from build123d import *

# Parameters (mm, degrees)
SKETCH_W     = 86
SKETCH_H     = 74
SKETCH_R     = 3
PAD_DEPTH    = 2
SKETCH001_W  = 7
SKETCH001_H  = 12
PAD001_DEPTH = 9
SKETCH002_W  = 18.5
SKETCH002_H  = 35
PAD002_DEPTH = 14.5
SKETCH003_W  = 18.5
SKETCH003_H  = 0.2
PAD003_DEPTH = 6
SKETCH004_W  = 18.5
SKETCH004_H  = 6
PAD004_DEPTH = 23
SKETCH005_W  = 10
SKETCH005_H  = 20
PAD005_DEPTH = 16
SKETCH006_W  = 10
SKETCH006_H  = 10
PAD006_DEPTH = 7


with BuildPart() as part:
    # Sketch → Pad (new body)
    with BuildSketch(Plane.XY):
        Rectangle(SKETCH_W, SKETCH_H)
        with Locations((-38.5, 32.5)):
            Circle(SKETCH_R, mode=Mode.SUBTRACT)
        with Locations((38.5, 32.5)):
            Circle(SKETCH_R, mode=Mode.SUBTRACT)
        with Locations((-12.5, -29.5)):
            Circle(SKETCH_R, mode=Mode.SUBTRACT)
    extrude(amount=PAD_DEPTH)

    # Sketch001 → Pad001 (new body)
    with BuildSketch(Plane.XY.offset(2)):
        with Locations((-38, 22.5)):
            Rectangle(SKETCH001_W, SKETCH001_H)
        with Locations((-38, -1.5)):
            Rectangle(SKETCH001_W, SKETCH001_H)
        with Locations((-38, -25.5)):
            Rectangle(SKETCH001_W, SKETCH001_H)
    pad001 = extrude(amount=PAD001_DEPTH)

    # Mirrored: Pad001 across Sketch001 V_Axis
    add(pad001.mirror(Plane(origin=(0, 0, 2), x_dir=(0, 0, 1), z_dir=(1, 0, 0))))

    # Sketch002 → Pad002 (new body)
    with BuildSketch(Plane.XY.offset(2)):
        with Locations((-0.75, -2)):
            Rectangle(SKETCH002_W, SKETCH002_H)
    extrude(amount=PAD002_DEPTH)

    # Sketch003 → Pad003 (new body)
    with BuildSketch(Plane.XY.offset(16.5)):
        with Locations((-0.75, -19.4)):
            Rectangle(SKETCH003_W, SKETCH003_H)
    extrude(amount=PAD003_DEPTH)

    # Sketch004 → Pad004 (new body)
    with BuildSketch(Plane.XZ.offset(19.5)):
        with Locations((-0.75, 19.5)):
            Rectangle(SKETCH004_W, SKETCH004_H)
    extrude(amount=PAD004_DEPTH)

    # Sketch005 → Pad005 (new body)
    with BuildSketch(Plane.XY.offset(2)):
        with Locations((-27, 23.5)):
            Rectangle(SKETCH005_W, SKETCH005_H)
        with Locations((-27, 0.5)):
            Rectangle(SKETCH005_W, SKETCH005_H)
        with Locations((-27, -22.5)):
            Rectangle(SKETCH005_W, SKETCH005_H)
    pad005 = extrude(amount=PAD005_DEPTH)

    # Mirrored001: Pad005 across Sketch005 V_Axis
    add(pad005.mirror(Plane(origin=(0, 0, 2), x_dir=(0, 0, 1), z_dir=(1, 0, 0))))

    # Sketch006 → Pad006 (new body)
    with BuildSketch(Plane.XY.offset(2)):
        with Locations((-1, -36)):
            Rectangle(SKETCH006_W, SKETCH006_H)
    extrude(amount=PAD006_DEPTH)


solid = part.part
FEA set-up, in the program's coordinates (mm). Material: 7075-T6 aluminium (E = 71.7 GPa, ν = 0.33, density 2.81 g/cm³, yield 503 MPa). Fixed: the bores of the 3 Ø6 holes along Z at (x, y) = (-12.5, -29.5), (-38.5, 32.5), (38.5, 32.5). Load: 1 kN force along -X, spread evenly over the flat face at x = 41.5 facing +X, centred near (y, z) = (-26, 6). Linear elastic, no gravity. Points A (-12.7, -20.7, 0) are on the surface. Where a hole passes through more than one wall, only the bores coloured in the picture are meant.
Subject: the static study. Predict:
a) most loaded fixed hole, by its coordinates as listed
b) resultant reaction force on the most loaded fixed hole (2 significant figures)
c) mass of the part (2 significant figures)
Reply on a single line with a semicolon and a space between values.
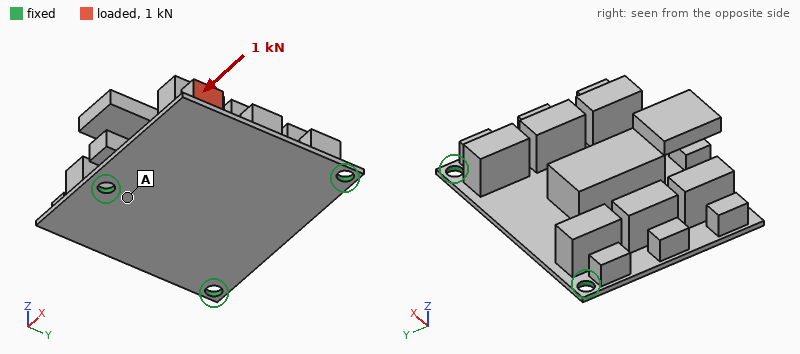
(-12.5, -29.5); 680 N; 140 g
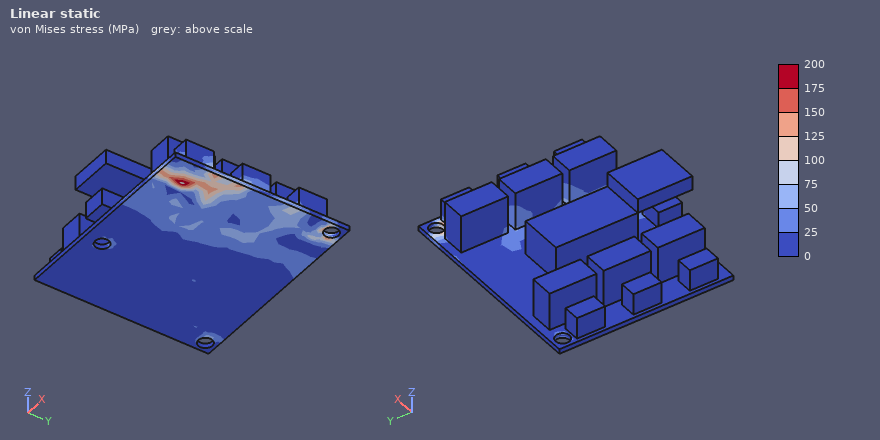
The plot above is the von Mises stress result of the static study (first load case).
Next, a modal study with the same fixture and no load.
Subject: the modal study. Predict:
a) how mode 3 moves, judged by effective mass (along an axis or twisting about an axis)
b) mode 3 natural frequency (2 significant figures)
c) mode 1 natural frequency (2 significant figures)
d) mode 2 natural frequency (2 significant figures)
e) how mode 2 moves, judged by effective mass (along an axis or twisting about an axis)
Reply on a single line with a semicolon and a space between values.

along Z; 1200 Hz; 660 Hz; 890 Hz; along Z
